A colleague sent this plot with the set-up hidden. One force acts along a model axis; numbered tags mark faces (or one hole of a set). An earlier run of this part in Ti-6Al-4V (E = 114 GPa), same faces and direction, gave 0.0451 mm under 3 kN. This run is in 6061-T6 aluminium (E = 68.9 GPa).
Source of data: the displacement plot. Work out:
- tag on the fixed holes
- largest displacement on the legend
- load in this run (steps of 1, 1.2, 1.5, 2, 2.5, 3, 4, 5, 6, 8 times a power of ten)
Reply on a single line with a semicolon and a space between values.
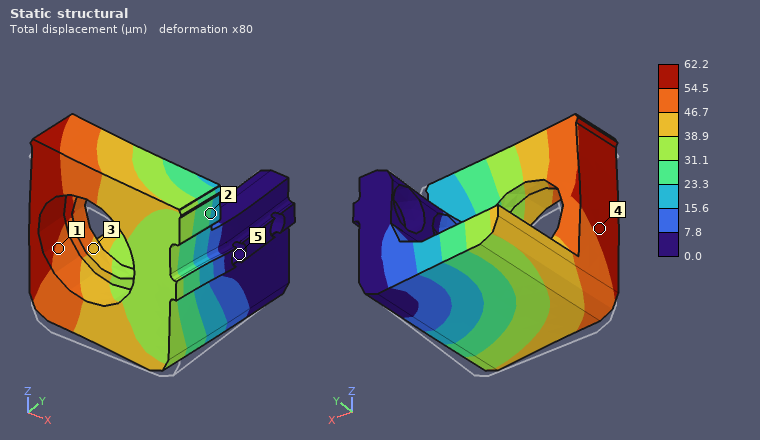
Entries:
5; 62.2 µm; 2.5 kN
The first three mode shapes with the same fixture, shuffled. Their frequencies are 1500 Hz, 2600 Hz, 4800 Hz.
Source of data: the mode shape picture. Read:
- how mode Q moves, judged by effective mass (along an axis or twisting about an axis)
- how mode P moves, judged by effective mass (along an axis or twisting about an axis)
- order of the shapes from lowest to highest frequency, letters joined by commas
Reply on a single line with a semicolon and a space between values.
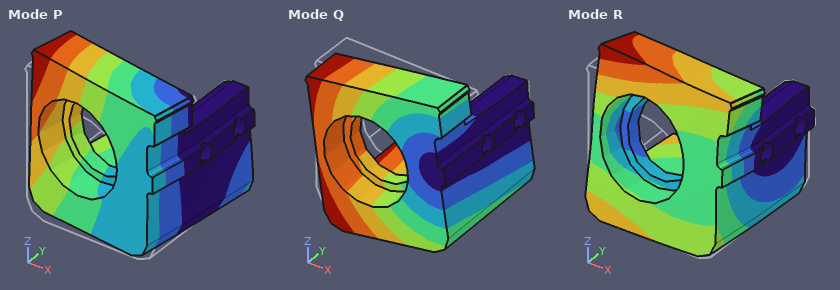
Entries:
along Z; along Y; Q, P, R
